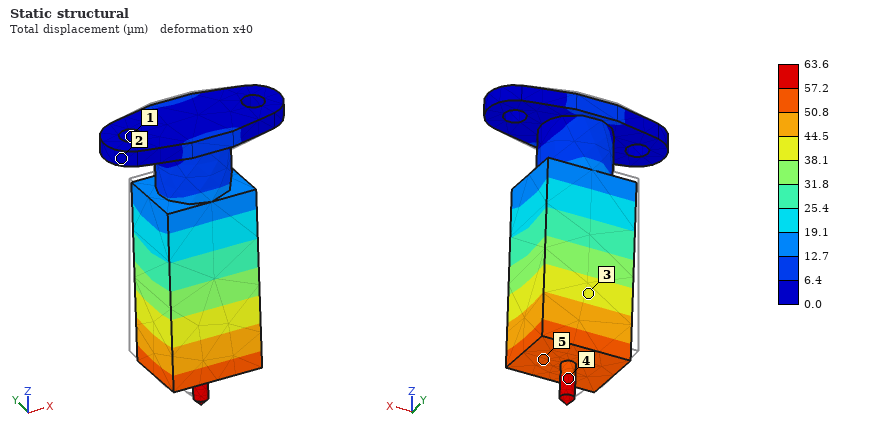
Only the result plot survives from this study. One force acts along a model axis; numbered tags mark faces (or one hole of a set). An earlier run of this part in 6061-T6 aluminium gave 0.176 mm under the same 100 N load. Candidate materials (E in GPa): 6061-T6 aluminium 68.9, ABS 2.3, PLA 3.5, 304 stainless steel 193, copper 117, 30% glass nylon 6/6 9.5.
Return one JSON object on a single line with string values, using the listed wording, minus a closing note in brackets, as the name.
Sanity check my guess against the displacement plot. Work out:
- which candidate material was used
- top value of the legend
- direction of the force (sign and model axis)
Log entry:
{"which candidate material was used": "304 stainless steel", "top value of the legend": "63.6 µm", "direction of the force": "-Y"}
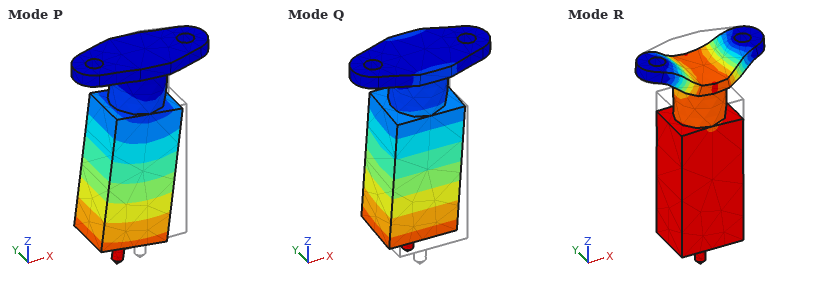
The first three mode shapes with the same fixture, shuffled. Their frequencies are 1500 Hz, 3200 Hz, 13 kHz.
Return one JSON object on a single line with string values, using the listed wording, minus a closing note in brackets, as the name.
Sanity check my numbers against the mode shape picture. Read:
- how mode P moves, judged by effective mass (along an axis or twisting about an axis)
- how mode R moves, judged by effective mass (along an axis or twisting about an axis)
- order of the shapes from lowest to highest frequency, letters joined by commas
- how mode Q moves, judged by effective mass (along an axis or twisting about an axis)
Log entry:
{"how mode P moves, judged by effective mass": "along X", "how mode R moves, judged by effective mass": "along Z", "order of the shapes from lowest to highest frequency, letters joined by commas": "Q, P, R", "how mode Q moves, judged by effective mass": "along Y"}
